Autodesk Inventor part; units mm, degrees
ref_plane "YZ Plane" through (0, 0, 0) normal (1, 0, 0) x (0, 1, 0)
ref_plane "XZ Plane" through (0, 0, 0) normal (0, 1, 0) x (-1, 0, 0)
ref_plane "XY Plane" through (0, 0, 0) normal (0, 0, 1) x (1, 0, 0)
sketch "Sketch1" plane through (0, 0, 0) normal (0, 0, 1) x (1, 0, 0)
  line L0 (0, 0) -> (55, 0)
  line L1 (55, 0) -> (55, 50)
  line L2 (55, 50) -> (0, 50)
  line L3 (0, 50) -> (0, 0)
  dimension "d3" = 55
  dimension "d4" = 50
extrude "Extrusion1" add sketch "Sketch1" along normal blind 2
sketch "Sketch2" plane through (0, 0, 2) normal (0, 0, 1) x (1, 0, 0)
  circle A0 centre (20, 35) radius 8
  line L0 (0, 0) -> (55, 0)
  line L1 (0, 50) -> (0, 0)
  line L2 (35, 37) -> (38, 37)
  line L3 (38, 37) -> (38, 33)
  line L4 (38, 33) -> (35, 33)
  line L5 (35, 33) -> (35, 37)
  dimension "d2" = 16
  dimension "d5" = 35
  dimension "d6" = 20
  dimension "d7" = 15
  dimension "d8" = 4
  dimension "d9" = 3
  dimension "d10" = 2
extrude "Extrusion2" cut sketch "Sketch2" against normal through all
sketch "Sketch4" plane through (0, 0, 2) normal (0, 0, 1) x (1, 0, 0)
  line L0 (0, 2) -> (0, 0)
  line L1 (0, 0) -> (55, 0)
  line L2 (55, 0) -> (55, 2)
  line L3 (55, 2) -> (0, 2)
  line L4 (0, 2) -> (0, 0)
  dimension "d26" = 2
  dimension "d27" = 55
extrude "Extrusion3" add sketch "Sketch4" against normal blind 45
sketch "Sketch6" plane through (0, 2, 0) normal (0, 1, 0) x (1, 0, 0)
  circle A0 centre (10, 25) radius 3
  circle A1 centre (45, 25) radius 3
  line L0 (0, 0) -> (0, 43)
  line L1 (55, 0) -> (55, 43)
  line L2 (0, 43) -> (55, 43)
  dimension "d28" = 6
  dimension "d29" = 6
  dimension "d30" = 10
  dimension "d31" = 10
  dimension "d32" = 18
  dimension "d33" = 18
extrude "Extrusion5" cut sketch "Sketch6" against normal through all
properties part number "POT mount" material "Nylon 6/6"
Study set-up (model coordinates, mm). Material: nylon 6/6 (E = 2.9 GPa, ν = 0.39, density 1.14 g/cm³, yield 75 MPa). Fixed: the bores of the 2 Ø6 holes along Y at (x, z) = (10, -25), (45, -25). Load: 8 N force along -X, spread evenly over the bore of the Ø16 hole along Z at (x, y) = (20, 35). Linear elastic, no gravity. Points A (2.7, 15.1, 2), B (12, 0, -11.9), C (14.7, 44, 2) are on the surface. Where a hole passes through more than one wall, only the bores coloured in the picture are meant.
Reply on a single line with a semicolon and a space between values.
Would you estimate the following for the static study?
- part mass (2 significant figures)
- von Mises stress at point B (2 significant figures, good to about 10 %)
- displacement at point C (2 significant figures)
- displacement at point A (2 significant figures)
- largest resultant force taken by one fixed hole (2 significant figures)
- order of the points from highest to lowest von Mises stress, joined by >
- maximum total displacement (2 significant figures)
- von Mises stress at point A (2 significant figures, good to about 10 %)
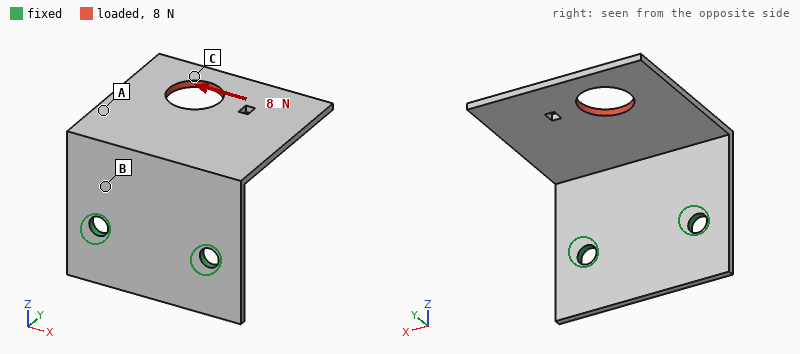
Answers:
11 g; 2.8 MPa; 0.67 mm; 0.45 mm; 9.7 N; B > A > C; 0.88 mm; 1.2 MPa
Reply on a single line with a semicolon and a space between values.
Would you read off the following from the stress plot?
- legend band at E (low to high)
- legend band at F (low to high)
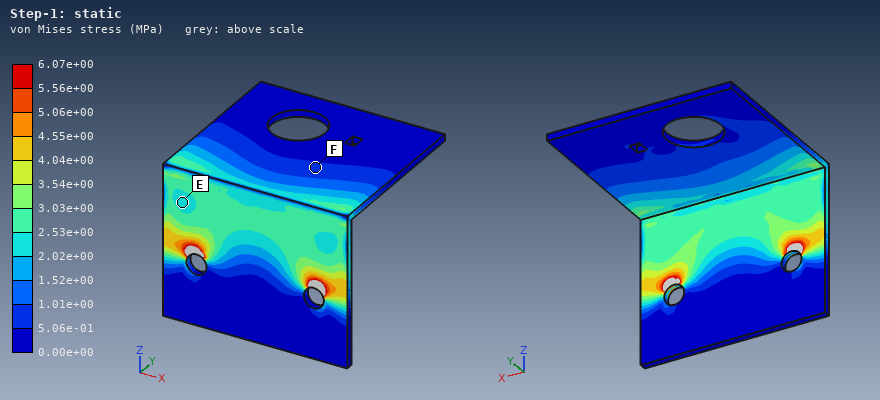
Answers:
2.02e+00 to 2.53e+00 MPa; 5.06e-01 to 1.01e+00 MPa
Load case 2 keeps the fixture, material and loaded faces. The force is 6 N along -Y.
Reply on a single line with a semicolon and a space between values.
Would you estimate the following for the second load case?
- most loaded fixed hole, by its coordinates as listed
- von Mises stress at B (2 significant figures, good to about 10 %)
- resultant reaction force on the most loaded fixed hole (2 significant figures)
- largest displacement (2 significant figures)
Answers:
(10, -25); 2.2 MPa; 4.2 N; 0.90 mm
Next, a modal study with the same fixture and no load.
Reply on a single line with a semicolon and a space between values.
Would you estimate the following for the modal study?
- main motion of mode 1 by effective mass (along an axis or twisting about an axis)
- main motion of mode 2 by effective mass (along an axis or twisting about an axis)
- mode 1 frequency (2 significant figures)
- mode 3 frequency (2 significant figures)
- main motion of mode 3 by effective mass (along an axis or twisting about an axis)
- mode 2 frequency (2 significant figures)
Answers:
along Z; along X; 130 Hz; 430 Hz; along Y; 260 Hz
